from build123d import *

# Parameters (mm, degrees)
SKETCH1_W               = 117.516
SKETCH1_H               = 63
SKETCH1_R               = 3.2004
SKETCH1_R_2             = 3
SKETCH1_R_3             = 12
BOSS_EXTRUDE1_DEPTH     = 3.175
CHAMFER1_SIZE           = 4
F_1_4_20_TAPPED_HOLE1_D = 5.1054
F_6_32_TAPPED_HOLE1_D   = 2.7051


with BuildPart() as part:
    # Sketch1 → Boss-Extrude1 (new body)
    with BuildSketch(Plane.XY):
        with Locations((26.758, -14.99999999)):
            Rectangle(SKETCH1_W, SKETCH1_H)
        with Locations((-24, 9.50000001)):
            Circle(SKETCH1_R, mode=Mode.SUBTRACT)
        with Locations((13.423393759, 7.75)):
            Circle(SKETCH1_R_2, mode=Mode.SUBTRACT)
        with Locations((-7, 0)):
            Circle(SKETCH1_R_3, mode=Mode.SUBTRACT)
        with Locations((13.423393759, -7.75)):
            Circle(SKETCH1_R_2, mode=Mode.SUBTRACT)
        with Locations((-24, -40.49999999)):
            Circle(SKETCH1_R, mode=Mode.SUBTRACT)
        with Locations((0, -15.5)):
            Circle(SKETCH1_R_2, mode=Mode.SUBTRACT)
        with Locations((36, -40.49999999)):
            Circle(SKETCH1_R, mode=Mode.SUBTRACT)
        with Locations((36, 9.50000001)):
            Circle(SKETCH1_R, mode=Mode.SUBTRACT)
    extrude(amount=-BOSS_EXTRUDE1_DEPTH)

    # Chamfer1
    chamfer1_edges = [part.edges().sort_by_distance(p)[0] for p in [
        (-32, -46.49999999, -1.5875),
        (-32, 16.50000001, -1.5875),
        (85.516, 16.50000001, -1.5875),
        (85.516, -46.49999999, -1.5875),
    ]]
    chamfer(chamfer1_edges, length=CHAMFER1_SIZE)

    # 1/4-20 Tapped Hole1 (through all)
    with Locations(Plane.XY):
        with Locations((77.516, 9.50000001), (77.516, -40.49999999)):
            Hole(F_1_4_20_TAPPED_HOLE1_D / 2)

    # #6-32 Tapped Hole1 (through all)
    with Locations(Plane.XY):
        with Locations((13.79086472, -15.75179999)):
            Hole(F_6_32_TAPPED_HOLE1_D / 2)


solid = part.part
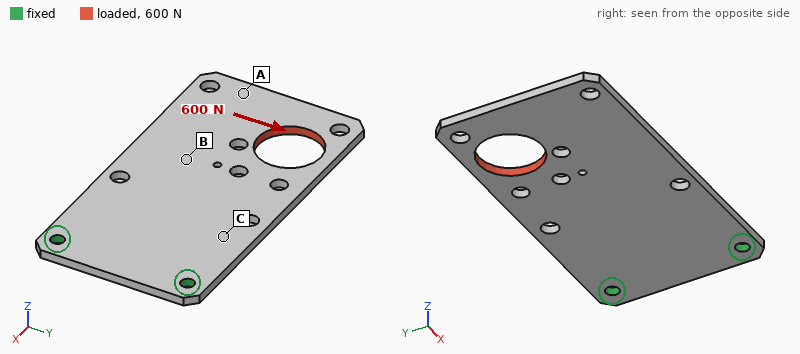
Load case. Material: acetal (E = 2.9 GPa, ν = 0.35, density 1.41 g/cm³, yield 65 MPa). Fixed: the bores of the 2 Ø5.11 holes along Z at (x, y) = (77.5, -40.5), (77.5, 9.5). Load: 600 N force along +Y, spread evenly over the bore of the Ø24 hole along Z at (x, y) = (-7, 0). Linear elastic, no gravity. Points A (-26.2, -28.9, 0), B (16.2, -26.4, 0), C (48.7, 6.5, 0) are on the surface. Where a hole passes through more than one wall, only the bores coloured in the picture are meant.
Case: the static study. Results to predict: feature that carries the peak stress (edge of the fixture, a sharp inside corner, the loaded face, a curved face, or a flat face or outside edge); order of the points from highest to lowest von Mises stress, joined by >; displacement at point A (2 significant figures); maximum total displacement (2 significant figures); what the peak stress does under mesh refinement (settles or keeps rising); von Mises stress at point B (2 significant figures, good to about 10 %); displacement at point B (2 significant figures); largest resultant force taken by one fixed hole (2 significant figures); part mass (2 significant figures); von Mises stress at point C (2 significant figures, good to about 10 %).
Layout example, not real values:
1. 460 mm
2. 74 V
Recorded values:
1. edge of the fixture
2. C > B > A
3. 1.4 mm
4. 1.5 mm
5. keeps rising
6. 6.0 MPa
7. 0.63 mm
8. 1.0 kN
9. 30 g
10. 12 MPa
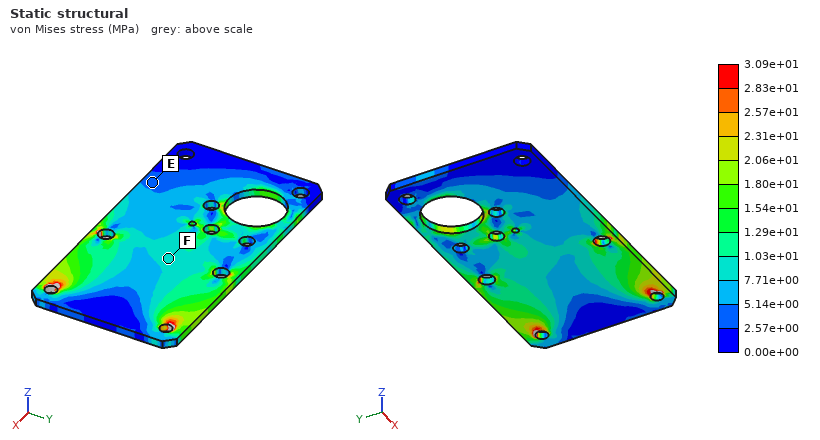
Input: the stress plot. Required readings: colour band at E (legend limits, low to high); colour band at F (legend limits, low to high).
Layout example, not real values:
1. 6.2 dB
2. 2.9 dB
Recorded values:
1. 2.57e+00 to 5.14e+00 MPa
2. 7.71e+00 to 1.03e+01 MPa
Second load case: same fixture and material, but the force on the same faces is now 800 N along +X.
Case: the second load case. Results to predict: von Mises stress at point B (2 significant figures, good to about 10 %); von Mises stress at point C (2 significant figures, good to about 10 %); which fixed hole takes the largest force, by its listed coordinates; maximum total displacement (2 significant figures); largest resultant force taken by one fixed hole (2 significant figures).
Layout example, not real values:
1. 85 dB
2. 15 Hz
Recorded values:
1. 3.0 MPa
2. 7.6 MPa
3. (77.5, 9.5)
4. 0.61 mm
5. 650 N
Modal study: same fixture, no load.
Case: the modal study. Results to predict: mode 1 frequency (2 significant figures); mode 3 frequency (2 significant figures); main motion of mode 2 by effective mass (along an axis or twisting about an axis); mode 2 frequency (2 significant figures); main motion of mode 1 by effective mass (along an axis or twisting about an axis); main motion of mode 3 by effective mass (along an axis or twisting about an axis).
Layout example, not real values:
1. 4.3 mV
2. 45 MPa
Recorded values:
1. 64 Hz
2. 360 Hz
3. twisting about X
4. 250 Hz
5. along Z
6. along Z
